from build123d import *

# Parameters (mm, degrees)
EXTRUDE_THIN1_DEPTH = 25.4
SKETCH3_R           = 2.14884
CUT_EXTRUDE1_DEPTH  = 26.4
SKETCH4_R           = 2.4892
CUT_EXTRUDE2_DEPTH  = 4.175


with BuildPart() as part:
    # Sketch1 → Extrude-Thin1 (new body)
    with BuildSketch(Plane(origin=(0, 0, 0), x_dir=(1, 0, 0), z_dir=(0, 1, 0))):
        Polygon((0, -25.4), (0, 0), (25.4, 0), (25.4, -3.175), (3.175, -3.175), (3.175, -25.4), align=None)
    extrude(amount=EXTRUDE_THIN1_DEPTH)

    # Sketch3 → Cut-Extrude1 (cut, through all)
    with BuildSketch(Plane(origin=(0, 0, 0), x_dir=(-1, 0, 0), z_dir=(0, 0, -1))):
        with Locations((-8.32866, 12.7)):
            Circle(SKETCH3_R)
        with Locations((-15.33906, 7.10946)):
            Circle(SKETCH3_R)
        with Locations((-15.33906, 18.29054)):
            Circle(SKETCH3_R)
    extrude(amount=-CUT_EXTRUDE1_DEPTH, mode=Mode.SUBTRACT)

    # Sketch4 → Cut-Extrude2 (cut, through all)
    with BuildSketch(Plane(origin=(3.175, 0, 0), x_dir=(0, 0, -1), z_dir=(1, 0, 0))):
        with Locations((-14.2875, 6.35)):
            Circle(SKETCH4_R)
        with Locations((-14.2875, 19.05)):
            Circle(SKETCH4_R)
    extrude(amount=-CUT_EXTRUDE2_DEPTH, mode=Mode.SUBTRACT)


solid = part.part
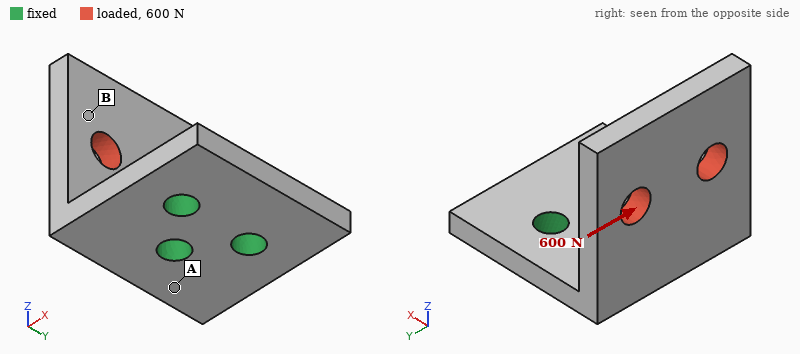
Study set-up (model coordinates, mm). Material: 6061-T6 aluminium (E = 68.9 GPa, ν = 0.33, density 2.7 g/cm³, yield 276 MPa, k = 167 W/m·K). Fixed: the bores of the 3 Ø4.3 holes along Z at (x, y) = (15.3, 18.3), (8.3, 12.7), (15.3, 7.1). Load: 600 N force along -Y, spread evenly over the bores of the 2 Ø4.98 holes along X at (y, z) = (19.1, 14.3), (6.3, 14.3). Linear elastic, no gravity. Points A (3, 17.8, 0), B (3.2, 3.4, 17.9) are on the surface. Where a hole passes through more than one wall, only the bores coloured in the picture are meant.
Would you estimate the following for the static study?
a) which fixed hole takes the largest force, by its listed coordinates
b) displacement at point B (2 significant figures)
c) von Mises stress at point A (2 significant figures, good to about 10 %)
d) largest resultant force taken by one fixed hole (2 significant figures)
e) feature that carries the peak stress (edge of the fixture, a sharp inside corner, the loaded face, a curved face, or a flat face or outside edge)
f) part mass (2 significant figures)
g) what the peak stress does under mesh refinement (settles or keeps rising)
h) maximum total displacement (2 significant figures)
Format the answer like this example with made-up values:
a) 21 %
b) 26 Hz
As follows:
a) (8.3, 12.7)
b) 0.10 mm
c) 45 MPa
d) 620 N
e) edge of the fixture
f) 9.7 g
g) keeps rising
h) 0.14 mm
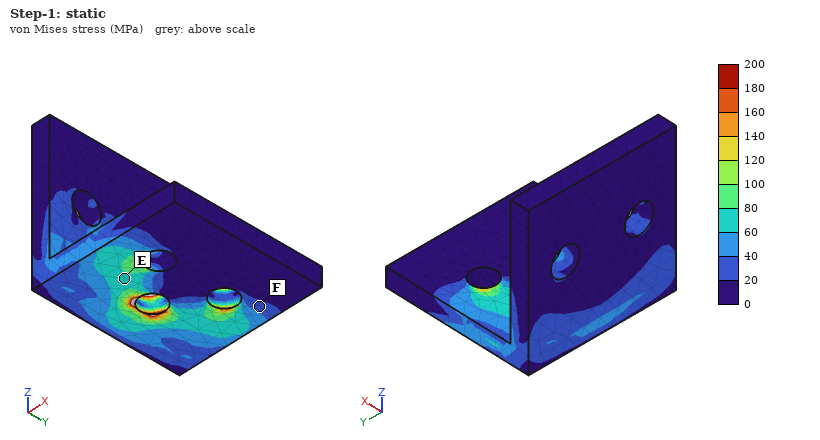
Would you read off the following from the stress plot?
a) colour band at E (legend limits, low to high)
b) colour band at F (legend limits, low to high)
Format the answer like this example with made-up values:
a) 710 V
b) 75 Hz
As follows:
a) 60 to 80 MPa
b) 20 to 40 MPa
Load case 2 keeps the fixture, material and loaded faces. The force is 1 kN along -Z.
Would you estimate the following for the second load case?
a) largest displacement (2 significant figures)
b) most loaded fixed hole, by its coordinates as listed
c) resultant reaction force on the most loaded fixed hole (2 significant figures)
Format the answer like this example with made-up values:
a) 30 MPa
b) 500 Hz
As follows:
a) 0.12 mm
b) (8.3, 12.7)
c) 1.2 kN
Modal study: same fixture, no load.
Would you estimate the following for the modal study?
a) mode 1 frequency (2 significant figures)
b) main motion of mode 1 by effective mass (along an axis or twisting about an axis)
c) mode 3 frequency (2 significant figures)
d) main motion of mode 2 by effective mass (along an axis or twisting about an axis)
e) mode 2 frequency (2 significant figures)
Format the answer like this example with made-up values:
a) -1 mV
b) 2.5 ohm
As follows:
a) 3300 Hz
b) along X
c) 9300 Hz
d) along Y
e) 5500 Hz
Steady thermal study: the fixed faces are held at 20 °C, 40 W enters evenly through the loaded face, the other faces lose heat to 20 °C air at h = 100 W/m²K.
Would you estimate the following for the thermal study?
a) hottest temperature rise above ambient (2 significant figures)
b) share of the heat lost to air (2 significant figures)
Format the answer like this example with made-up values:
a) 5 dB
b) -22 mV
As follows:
a) 57 K
b) 16 %
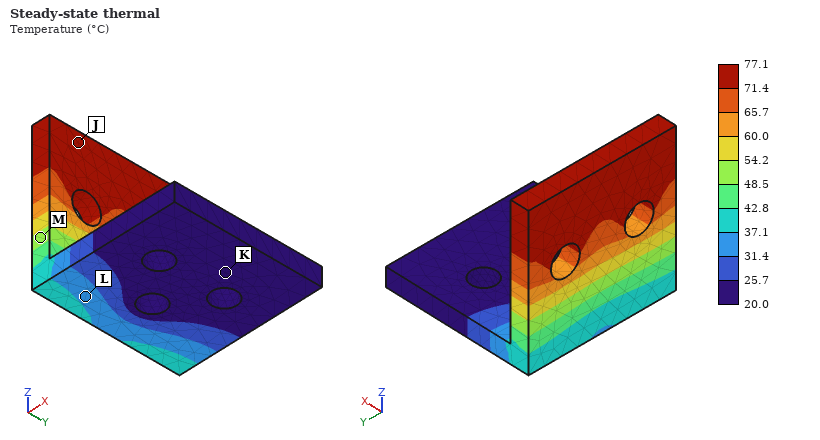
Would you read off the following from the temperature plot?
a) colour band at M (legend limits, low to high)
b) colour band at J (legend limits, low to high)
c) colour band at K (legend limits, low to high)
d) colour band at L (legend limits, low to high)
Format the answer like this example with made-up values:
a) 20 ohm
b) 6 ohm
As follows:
a) 48.5 to 54.2 °C
b) 71.4 to 77.1 °C
c) 20.0 to 25.7 °C
d) 31.4 to 37.1 °C
